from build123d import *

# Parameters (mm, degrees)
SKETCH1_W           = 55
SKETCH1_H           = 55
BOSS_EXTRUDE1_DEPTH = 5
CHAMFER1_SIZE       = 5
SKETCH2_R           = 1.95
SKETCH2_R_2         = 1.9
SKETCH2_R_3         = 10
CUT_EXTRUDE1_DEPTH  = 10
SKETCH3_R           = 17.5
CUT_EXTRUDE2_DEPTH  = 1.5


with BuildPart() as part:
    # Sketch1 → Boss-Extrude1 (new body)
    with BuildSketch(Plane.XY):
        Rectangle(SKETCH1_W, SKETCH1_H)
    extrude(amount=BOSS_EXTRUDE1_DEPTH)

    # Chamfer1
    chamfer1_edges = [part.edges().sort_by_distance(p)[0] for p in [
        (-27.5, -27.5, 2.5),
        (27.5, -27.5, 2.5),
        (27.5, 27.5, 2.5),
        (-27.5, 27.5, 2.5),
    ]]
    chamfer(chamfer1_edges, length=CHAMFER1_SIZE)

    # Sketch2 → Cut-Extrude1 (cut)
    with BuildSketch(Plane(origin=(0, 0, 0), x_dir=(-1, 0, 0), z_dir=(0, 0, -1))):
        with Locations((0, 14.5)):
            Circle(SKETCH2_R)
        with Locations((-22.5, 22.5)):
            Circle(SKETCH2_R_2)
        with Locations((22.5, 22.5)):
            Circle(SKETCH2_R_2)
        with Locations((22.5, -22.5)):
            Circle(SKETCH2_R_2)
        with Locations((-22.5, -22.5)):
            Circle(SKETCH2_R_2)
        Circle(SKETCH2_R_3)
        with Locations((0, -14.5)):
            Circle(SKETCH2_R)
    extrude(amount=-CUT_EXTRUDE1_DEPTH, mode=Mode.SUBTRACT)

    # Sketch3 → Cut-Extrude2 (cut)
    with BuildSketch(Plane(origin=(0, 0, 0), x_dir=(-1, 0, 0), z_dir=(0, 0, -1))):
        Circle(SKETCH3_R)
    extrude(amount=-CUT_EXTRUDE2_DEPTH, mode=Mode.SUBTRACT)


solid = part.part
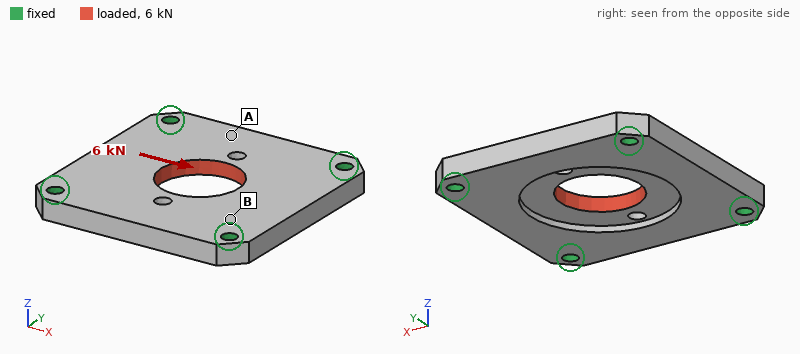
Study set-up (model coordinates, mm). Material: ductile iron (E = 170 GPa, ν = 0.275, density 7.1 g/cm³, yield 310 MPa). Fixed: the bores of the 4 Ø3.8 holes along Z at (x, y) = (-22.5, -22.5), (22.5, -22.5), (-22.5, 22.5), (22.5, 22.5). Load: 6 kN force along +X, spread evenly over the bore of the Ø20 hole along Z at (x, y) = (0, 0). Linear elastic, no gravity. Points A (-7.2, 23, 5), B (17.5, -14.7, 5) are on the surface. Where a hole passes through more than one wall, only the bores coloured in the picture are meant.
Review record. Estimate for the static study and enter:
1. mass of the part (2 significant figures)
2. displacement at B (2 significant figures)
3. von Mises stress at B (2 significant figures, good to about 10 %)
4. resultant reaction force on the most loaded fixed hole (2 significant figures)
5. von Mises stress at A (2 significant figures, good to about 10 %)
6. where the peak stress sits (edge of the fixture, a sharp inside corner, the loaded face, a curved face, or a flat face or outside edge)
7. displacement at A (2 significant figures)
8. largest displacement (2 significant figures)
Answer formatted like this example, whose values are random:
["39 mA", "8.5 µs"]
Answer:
["85 g", "2.4 µm", "31 MPa", "1.6 kN", "9.9 MPa", "a flat face or outside edge", "1.5 µm", "6.6 µm"]
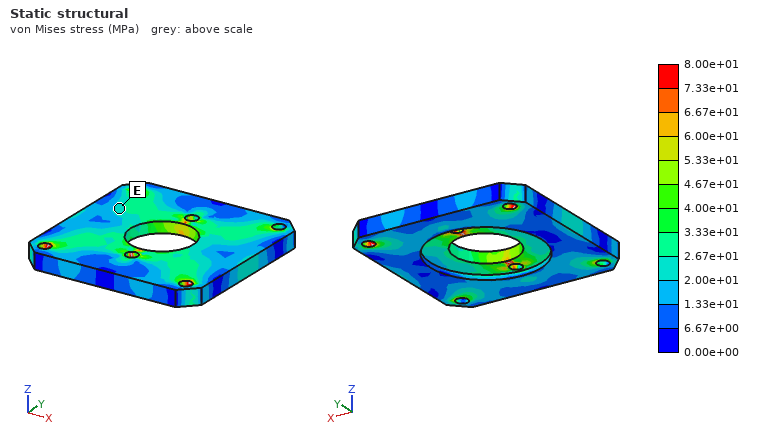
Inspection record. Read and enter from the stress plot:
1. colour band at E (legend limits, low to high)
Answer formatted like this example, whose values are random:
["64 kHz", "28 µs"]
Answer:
["2.00e+01 to 2.67e+01 MPa"]
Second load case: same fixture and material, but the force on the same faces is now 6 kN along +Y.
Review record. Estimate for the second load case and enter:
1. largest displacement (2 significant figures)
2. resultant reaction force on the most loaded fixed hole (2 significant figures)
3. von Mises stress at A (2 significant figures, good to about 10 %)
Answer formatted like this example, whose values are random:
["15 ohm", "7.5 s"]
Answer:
["6.8 µm", "1.6 kN", "15 MPa"]
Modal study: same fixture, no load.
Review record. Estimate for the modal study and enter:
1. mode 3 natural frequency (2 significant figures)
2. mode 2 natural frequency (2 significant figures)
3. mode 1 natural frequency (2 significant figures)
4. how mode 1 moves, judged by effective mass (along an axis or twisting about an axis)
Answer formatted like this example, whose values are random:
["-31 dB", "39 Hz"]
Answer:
["12 kHz", "12 kHz", "8800 Hz", "along Z"]
